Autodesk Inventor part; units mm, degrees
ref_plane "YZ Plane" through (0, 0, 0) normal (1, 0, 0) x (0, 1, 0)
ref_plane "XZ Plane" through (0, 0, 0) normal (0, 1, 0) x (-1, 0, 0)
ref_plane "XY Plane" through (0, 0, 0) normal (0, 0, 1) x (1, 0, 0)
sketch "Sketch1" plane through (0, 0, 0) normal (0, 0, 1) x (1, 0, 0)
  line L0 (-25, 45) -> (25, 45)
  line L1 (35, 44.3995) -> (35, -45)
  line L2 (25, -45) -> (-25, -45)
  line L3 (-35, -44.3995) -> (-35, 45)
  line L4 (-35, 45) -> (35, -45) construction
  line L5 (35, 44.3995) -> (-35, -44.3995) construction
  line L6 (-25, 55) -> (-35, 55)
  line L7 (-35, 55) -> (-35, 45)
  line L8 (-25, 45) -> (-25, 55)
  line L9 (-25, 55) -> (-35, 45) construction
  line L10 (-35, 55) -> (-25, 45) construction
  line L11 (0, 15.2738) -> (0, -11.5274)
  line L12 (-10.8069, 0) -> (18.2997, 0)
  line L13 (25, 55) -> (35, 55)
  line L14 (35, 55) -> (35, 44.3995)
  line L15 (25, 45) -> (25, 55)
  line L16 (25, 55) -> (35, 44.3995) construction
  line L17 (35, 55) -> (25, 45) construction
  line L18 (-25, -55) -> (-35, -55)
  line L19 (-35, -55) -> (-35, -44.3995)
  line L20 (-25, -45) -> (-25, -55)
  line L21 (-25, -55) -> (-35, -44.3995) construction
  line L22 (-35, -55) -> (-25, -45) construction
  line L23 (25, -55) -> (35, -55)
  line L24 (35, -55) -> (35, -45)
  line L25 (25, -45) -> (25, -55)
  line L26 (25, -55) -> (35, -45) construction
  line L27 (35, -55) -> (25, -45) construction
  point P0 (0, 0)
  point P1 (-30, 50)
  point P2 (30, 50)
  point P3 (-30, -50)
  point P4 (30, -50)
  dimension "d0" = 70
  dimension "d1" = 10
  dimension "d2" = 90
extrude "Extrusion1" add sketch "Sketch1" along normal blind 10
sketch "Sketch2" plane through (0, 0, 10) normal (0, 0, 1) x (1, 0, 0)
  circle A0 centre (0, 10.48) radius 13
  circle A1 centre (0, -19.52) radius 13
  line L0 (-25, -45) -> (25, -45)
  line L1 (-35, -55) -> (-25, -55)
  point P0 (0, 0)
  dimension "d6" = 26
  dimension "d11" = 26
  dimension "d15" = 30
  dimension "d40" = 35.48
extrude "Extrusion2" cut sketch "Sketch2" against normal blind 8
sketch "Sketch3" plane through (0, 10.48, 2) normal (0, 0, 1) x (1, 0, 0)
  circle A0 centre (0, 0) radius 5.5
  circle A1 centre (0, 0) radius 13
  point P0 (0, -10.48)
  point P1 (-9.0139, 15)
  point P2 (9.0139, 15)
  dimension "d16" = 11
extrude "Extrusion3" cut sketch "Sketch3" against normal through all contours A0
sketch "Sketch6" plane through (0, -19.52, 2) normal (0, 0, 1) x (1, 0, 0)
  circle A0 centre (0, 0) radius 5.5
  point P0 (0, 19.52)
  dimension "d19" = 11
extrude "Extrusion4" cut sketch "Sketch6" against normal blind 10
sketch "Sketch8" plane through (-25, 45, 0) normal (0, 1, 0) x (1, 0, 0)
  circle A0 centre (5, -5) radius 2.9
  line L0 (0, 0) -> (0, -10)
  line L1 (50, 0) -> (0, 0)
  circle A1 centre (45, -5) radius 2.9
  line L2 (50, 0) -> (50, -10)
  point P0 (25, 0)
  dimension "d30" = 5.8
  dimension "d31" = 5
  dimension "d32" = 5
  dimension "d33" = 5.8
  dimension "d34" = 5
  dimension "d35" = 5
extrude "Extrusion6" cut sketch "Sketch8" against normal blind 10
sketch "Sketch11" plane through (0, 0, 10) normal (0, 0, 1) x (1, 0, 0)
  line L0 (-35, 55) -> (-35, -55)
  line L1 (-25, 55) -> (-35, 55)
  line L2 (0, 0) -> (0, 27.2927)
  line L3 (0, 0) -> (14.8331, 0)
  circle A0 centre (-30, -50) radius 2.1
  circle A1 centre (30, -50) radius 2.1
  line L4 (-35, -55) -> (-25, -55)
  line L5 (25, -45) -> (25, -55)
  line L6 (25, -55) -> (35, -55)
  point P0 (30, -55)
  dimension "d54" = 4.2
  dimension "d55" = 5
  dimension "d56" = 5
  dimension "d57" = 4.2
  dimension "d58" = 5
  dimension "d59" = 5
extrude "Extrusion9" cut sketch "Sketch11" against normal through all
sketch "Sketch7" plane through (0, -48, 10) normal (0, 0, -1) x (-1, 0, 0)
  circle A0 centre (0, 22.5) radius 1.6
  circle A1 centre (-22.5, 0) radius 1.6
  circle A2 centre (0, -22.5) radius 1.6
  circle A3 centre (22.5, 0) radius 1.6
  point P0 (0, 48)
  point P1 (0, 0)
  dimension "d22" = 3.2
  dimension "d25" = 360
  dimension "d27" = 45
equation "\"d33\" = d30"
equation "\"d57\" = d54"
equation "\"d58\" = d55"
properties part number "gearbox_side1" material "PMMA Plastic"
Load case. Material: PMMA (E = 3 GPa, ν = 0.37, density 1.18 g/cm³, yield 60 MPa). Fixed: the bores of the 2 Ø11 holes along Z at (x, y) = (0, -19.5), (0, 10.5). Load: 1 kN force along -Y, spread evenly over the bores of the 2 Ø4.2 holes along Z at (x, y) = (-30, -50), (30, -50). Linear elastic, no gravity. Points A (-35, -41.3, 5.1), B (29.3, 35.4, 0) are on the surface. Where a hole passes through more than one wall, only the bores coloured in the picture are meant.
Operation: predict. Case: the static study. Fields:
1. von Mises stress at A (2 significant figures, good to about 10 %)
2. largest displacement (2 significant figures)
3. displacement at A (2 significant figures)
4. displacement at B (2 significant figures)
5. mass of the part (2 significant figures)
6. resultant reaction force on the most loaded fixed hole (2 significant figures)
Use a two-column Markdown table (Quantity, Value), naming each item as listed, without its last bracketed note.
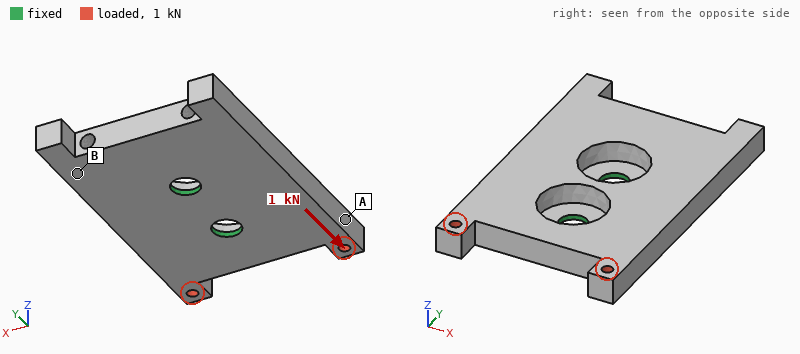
| Quantity | Value |
|---|---|
| von Mises stress at A | 6.2 MPa |
| largest displacement | 0.26 mm |
| displacement at A | 0.19 mm |
| displacement at B | 0.15 mm |
| mass of the part | 68 g |
| resultant reaction force on the most loaded fixed hole | 520 N |
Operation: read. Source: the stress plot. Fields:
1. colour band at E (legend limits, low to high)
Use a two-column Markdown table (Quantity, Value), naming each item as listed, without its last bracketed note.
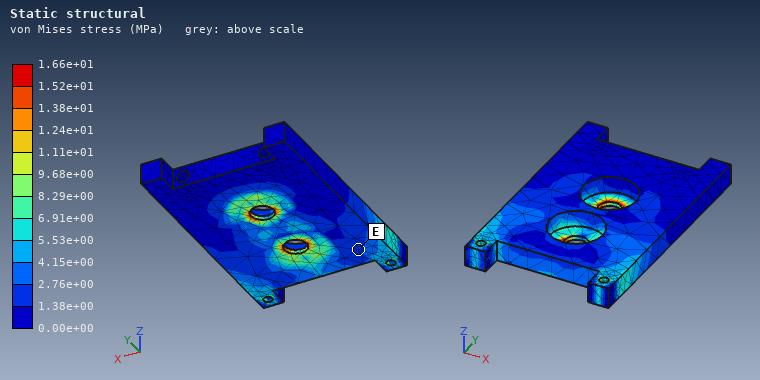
| Quantity | Value |
|---|---|
| colour band at E | 1.38e+00 to 2.76e+00 MPa |
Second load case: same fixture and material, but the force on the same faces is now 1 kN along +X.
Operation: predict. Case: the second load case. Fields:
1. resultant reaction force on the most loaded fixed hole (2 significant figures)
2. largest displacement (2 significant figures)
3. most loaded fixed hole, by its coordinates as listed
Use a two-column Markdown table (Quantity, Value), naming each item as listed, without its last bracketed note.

| Quantity | Value |
|---|---|
| resultant reaction force on the most loaded fixed hole | 1.7 kN |
| largest displacement | 1.2 mm |
| most loaded fixed hole, by its coordinates as listed | (0, -19.5) |
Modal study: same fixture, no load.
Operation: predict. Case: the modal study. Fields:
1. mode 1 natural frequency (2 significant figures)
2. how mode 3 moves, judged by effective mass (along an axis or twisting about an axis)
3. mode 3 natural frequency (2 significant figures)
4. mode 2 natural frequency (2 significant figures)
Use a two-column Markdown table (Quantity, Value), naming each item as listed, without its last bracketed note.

| Quantity | Value |
|---|---|
| mode 1 natural frequency | 400 Hz |
| how mode 3 moves, judged by effective mass | along Z |
| mode 3 natural frequency | 1100 Hz |
| mode 2 natural frequency | 670 Hz |
